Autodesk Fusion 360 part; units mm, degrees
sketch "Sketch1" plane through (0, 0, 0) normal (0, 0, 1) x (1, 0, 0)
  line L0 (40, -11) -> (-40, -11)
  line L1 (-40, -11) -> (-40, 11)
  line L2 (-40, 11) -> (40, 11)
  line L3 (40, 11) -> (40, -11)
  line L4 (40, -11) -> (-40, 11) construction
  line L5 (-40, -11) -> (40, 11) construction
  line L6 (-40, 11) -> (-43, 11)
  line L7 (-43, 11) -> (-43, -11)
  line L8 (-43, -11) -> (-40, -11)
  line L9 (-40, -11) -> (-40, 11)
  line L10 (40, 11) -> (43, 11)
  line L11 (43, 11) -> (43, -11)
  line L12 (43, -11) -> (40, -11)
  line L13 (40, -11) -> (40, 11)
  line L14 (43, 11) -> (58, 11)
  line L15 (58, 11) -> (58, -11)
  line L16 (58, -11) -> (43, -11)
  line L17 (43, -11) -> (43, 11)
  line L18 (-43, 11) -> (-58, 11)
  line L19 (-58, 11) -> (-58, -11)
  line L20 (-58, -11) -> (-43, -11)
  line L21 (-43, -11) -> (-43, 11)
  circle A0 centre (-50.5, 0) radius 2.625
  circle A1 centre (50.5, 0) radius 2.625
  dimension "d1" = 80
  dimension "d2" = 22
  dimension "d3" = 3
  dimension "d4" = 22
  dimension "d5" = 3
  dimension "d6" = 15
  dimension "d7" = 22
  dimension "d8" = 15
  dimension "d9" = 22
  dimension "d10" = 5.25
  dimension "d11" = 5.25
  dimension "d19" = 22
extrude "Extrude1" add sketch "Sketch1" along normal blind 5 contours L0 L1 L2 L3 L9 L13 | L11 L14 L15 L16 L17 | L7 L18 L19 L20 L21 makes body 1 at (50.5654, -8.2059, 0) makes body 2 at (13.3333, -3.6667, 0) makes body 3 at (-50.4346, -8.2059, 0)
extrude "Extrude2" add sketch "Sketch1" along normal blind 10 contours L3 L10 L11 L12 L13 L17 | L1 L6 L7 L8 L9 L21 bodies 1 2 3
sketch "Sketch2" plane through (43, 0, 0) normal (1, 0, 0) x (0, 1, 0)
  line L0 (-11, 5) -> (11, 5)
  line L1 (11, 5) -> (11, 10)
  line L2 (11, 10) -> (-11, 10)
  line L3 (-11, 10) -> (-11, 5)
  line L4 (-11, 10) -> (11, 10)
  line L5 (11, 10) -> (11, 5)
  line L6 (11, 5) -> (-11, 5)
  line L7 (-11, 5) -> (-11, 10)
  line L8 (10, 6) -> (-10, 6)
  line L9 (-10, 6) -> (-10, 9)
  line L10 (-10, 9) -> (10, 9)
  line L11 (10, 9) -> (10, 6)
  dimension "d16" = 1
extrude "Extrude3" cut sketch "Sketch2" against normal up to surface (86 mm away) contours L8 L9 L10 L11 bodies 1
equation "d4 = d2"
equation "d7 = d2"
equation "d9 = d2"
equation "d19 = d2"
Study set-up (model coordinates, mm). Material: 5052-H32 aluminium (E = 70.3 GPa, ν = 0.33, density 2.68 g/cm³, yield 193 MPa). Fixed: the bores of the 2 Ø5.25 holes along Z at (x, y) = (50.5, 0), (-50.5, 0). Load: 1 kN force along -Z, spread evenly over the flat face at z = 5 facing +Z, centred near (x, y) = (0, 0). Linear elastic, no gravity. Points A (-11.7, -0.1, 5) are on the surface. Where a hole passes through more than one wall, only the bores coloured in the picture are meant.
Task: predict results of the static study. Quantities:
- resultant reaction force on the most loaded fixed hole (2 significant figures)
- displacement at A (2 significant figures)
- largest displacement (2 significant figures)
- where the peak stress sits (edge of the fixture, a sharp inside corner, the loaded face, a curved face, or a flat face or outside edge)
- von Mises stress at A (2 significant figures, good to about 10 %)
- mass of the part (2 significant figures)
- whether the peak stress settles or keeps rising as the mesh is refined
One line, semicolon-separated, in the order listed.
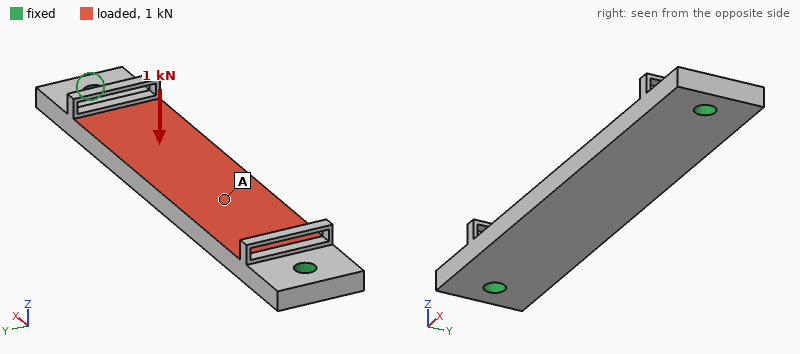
500 N; 0.18 mm; 0.20 mm; edge of the fixture; 44 MPa; 34 g; keeps rising
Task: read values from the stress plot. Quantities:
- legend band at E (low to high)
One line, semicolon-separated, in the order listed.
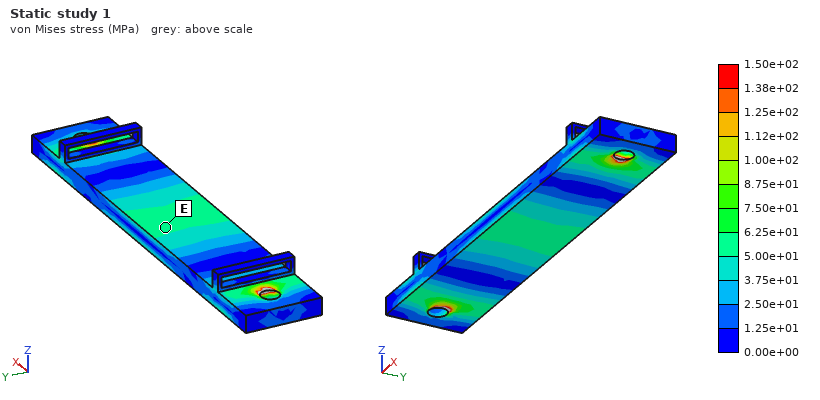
5.00e+01 to 6.25e+01 MPa
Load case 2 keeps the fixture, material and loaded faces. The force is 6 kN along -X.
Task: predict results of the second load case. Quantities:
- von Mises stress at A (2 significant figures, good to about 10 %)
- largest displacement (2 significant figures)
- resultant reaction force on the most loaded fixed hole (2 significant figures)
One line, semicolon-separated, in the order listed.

11 MPa; 14 µm; 3.0 kN
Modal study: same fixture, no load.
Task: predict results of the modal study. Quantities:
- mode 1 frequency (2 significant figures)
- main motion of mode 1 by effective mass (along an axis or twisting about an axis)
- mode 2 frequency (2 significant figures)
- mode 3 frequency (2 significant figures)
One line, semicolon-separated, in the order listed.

2600 Hz; along Z; 6600 Hz; 6700 Hz
